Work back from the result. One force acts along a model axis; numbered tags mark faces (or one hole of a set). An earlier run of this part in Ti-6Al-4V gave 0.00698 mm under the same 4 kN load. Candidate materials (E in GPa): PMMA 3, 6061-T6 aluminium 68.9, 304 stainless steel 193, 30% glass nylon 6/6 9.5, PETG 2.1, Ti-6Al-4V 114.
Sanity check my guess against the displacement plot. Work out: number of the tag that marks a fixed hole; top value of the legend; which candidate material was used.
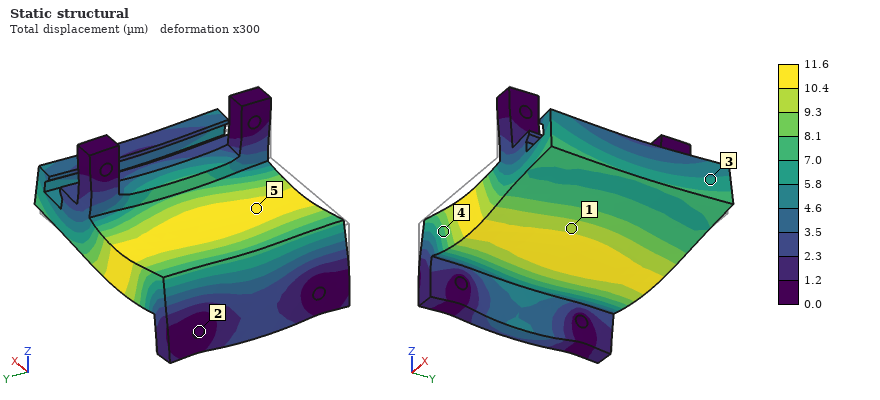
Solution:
2
11.6 µm
6061-T6 aluminium
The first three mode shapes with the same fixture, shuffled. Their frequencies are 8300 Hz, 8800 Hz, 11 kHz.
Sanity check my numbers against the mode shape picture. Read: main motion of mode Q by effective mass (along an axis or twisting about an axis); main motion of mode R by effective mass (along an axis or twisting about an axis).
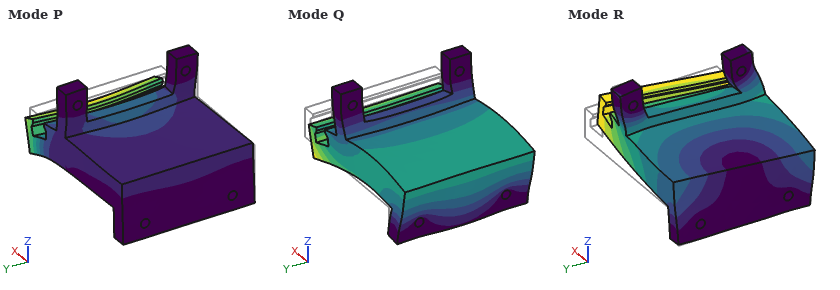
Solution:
along X
along Y
